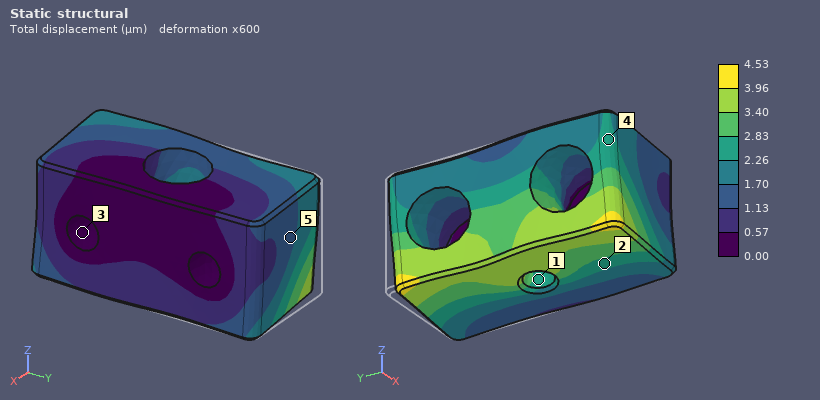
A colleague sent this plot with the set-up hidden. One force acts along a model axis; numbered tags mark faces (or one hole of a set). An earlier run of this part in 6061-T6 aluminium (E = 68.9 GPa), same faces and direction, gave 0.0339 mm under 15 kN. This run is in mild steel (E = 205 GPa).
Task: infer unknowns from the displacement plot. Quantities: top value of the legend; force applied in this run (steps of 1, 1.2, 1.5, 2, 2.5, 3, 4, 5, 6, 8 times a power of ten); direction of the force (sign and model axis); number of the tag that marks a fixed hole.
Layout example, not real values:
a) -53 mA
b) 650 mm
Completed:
a) 4.53 µm
b) 6 kN
c) -Y
d) 3
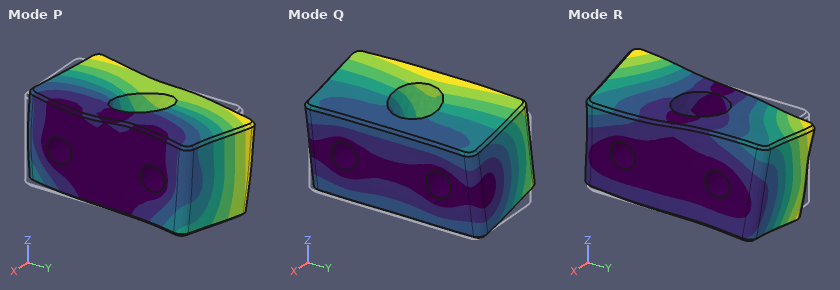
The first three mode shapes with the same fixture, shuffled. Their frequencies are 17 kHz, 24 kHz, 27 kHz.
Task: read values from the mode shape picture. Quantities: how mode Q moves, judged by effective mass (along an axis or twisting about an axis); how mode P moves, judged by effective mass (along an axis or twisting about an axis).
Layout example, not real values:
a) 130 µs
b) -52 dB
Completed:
a) along Z
b) along Y
